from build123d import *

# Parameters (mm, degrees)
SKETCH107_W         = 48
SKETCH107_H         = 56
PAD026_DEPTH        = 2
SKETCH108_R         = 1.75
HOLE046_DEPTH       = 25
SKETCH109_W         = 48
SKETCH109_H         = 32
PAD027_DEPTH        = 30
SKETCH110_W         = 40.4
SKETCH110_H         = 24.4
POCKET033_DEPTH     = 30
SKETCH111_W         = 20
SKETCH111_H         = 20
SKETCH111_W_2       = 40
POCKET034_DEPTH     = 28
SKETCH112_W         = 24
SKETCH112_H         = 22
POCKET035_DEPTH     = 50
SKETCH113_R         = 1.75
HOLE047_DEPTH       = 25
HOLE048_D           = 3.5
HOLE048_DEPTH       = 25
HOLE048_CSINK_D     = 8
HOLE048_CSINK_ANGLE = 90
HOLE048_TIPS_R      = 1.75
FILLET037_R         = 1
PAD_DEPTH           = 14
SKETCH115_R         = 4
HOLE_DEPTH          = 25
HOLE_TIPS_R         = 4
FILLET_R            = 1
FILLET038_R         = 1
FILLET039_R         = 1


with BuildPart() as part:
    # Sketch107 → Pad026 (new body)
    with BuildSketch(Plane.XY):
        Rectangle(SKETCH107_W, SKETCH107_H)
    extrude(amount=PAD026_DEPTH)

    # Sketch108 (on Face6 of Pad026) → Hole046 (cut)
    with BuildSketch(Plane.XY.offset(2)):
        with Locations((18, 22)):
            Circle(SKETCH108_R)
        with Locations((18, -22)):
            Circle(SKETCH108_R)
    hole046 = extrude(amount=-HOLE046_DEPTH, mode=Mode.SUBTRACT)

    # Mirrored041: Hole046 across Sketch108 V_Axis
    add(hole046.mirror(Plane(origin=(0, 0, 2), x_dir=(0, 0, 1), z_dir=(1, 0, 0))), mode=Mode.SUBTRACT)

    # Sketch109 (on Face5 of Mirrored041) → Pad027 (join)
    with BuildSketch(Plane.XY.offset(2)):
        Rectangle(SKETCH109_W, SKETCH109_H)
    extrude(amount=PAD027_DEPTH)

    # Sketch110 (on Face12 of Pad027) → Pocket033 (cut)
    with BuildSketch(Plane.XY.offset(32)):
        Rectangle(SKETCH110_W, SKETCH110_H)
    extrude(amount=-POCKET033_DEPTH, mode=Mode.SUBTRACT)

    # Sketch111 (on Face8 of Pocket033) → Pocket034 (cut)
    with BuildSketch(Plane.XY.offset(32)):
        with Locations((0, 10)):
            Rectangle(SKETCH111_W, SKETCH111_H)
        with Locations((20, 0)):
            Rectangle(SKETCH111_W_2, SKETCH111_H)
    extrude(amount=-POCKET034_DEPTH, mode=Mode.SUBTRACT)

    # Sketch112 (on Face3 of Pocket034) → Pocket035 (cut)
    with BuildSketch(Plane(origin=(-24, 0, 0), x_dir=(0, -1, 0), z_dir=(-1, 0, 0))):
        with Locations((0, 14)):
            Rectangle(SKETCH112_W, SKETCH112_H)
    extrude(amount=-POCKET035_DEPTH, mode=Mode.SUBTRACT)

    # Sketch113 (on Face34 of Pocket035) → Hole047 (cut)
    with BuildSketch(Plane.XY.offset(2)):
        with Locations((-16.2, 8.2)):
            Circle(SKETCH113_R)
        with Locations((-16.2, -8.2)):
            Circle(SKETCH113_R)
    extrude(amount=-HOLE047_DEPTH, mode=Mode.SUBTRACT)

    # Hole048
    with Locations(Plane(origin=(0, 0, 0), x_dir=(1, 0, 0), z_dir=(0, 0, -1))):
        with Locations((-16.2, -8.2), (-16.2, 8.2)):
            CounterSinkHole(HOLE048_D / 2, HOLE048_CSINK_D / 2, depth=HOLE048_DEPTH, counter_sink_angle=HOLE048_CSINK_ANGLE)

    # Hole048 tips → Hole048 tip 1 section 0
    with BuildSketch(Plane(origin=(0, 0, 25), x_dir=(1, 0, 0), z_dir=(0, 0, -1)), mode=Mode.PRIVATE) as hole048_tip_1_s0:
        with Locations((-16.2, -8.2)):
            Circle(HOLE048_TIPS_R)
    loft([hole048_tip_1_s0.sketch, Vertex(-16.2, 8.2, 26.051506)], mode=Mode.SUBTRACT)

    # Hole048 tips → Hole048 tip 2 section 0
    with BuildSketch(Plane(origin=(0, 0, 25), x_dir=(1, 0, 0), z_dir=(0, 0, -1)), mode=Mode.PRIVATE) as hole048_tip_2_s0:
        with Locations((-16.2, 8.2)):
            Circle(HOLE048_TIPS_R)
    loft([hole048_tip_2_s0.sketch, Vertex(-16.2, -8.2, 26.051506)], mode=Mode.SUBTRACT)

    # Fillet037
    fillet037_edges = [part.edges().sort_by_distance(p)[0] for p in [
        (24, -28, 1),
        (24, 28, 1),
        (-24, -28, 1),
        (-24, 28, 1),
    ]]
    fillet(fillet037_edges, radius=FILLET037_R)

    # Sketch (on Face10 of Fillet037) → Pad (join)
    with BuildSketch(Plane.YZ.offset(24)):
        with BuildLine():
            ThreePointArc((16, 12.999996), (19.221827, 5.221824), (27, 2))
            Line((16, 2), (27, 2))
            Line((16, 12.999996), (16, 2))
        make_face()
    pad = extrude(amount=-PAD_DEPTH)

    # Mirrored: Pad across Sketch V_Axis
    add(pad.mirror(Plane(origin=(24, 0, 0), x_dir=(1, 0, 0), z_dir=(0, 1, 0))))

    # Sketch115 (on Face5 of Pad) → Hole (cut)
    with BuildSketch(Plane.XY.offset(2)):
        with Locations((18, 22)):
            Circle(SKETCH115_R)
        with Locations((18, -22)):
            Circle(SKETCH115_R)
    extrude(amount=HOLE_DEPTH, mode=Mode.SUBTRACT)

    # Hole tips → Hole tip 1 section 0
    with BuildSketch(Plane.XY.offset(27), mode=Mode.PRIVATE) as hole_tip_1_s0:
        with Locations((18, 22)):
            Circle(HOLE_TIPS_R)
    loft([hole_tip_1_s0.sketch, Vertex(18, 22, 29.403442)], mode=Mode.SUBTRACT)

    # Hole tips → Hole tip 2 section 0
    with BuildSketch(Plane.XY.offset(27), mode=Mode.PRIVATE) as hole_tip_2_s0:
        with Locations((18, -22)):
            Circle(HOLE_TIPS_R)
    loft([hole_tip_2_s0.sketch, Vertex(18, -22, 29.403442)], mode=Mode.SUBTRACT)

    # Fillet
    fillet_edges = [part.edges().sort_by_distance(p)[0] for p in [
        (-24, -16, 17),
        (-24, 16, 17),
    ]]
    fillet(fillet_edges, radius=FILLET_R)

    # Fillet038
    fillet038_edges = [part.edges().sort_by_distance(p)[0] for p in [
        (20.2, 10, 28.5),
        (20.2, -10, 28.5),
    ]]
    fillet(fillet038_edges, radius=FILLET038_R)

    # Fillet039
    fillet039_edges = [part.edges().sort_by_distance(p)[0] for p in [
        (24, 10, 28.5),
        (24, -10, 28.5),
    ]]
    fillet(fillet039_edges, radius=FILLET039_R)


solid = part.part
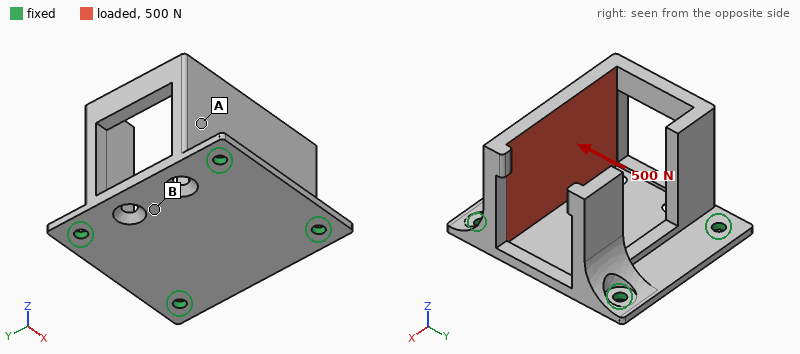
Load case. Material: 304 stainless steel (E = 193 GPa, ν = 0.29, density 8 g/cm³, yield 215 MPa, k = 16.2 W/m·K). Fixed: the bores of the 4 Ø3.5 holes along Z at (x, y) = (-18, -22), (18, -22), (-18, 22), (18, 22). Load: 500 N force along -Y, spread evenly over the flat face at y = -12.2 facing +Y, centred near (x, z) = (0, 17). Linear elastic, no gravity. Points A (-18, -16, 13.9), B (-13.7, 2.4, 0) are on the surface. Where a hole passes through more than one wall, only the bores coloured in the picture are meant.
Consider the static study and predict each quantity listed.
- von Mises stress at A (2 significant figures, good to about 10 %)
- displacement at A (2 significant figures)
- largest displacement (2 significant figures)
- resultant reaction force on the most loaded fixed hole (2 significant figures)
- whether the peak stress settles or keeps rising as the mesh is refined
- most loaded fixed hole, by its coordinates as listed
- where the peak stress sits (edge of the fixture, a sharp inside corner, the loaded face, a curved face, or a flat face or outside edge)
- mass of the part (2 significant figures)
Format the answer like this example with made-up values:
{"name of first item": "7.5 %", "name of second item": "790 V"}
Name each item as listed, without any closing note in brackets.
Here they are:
{"von Mises stress at A": "13 MPa", "displacement at A": "13 µm", "largest displacement": "57 µm", "resultant reaction force on the most loaded fixed hole": "210 N", "whether the peak stress settles or keeps rising as the mesh is refined": "keeps rising", "most loaded fixed hole, by its coordinates as listed": "(18, -22)", "where the peak stress sits": "edge of the fixture", "mass of the part": "120 g"}
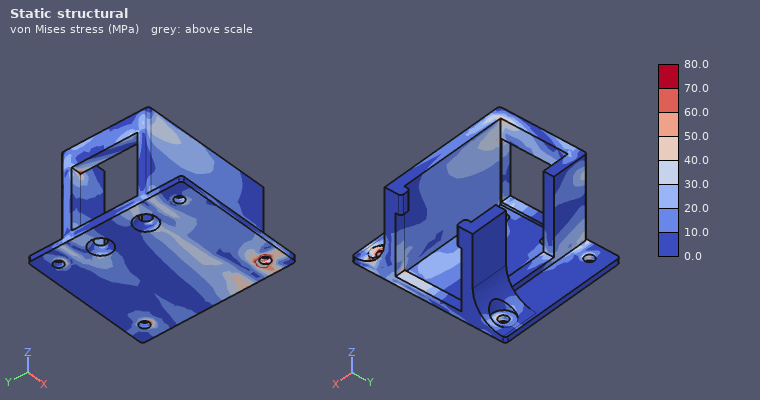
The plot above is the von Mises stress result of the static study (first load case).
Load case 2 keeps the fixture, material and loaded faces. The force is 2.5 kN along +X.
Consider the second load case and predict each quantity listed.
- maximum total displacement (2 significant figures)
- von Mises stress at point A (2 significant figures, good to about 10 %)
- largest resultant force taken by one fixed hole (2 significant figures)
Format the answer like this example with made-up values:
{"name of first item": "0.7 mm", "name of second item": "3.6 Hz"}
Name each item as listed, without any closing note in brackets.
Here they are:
{"maximum total displacement": "49 µm", "von Mises stress at point A": "29 MPa", "largest resultant force taken by one fixed hole": "1.6 kN"}
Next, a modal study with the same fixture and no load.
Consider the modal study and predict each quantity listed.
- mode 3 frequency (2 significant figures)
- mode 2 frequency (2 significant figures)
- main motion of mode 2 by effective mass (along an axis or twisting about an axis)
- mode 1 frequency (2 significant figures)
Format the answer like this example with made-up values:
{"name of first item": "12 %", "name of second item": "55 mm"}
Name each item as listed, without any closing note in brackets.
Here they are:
{"mode 3 frequency": "3500 Hz", "mode 2 frequency": "3000 Hz", "main motion of mode 2 by effective mass": "along Y", "mode 1 frequency": "2500 Hz"}
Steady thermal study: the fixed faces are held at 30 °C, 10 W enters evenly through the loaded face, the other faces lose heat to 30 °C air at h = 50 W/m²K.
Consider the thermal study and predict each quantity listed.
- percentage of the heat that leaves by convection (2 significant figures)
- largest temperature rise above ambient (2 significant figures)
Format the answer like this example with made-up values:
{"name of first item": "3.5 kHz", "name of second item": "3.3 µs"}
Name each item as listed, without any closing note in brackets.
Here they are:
{"percentage of the heat that leaves by convection": "66 %", "largest temperature rise above ambient": "46 K"}
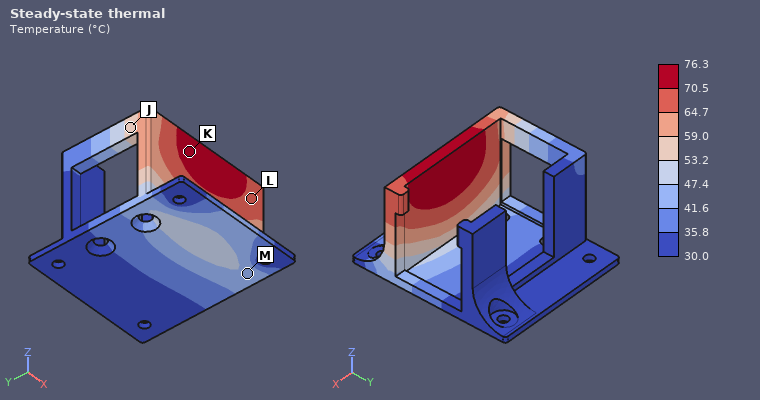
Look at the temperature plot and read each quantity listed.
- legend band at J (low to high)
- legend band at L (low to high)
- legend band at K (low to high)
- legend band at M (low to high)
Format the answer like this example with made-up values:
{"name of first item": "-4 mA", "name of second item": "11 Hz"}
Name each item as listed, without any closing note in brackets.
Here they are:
{"legend band at J": "53.2 to 59.0 °C", "legend band at L": "64.7 to 70.5 °C", "legend band at K": "70.5 to 76.3 °C", "legend band at M": "41.6 to 47.4 °C"}
